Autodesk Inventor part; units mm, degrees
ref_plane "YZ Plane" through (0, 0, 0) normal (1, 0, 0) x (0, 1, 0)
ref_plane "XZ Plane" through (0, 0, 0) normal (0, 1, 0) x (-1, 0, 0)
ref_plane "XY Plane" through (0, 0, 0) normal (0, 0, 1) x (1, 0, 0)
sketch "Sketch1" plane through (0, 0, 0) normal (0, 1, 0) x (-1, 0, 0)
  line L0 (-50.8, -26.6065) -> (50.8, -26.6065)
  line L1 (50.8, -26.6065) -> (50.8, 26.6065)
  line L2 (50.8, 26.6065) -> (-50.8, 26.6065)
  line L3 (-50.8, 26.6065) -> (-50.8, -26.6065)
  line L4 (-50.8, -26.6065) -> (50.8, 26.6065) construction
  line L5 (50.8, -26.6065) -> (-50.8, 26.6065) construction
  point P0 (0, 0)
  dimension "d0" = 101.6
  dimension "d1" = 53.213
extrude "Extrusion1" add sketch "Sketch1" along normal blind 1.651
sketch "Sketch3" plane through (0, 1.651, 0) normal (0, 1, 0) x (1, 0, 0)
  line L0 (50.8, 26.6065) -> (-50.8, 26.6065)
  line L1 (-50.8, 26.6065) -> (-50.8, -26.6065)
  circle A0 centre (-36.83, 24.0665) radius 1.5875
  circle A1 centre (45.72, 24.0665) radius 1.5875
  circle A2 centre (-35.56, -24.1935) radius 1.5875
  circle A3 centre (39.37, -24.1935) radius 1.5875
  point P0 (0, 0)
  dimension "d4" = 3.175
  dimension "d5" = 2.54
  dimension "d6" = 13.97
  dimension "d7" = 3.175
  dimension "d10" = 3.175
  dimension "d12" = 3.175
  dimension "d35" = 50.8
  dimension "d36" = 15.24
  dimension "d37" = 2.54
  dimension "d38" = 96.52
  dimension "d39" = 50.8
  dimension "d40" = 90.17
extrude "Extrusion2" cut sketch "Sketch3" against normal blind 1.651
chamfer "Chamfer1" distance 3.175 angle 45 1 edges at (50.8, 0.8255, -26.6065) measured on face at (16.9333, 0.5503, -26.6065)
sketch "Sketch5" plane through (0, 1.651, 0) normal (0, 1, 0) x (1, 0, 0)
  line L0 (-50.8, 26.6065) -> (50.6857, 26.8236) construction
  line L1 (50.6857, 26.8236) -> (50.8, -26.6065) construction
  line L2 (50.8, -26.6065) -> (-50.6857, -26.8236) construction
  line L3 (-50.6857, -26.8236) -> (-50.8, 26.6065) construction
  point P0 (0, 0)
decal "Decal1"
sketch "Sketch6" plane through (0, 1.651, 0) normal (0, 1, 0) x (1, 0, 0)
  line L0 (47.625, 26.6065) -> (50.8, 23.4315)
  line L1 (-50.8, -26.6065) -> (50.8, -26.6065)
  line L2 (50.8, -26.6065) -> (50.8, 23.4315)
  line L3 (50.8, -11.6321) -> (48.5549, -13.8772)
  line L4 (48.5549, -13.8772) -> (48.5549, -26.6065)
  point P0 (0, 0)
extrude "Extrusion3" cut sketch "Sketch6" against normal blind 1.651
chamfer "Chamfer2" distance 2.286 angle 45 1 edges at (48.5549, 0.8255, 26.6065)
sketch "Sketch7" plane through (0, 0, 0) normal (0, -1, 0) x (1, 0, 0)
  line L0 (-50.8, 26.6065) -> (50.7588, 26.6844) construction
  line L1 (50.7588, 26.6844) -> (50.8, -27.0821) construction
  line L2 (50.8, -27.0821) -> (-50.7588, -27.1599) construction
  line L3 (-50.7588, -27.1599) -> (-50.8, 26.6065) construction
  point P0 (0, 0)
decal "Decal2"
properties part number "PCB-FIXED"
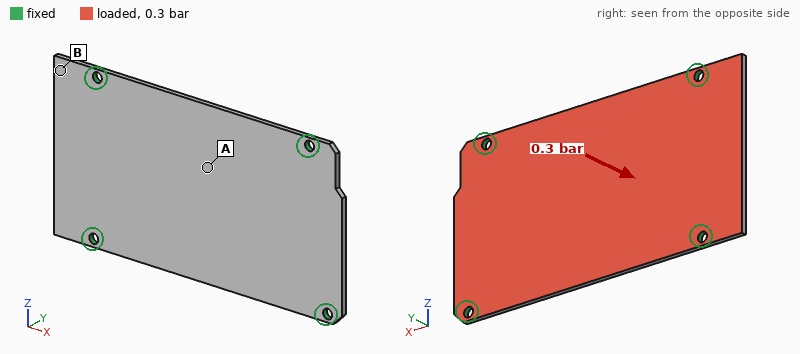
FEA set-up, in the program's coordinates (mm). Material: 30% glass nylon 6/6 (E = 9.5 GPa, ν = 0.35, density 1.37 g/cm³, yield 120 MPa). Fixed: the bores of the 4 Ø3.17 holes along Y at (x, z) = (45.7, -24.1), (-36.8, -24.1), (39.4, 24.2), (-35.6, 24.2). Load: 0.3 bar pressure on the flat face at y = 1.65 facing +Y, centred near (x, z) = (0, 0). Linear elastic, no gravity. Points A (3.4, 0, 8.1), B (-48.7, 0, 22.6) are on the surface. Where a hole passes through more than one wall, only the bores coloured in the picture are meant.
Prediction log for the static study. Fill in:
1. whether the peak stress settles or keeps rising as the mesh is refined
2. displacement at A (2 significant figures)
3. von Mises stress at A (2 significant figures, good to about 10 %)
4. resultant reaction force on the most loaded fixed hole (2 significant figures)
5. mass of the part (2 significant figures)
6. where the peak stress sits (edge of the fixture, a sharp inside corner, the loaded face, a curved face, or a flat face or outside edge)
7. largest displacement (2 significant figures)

keeps rising
1.1 mm
17 MPa
44 N
12 g
edge of the fixture
1.3 mm
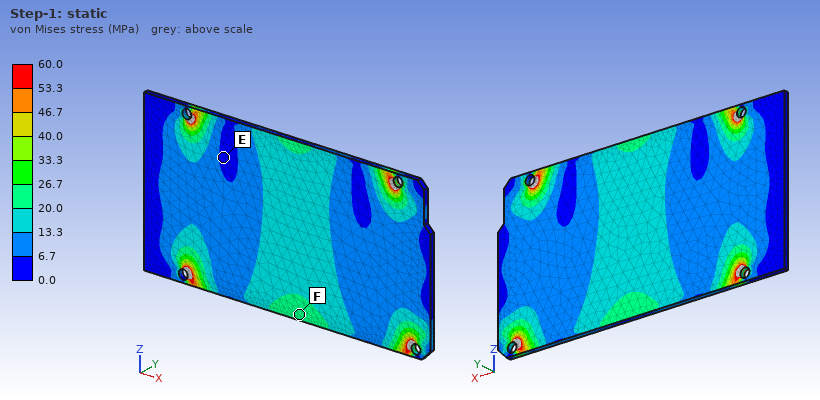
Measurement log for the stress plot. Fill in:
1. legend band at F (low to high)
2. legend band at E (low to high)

20.0 to 26.7 MPa
0.0 to 6.7 MPa
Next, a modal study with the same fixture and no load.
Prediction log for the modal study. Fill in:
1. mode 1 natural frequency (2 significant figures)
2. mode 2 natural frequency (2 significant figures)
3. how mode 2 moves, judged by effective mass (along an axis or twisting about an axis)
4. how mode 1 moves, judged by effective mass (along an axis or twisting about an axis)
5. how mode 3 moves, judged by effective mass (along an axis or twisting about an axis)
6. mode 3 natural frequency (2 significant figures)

610 Hz
1000 Hz
twisting about X
along Y
twisting about Z
1600 Hz
